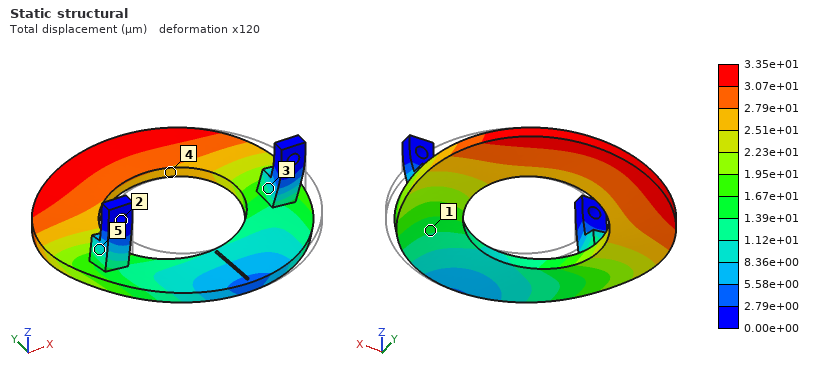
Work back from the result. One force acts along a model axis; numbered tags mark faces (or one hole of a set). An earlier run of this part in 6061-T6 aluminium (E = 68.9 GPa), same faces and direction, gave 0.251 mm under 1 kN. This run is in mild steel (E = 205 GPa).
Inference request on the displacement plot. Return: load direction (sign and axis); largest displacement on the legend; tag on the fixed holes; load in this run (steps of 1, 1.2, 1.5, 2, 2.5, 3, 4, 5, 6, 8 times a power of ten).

-X
3.35e+01 µm
2
400 N
